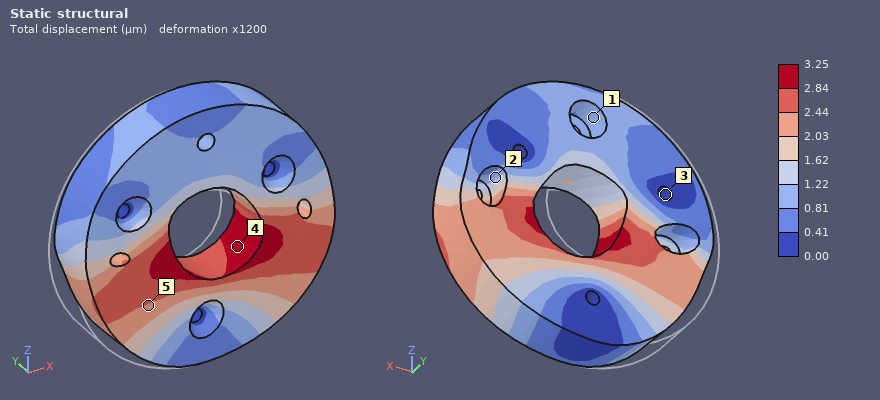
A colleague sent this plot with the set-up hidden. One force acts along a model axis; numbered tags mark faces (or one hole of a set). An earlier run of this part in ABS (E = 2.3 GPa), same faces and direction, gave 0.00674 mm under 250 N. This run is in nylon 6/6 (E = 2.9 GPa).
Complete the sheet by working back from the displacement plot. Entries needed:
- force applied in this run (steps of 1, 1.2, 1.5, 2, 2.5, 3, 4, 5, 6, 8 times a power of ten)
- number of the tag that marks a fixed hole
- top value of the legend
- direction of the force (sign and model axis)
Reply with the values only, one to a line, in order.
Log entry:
150 N
3
3.25 µm
+X
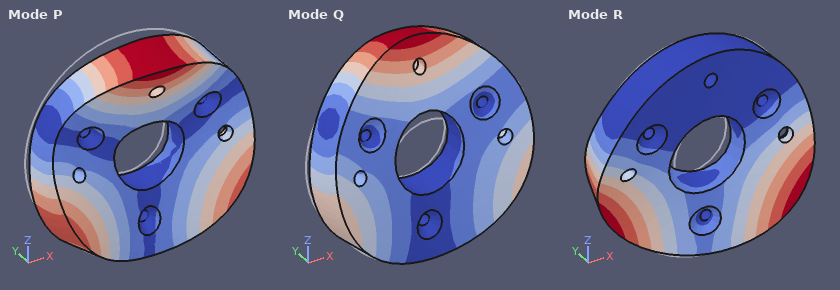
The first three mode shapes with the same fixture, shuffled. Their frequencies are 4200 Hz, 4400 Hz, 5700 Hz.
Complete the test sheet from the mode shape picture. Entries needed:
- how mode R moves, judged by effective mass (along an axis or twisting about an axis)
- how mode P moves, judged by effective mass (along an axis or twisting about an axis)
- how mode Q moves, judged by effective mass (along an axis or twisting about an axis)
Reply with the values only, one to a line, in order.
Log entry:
twisting about Z
along Y
twisting about X
